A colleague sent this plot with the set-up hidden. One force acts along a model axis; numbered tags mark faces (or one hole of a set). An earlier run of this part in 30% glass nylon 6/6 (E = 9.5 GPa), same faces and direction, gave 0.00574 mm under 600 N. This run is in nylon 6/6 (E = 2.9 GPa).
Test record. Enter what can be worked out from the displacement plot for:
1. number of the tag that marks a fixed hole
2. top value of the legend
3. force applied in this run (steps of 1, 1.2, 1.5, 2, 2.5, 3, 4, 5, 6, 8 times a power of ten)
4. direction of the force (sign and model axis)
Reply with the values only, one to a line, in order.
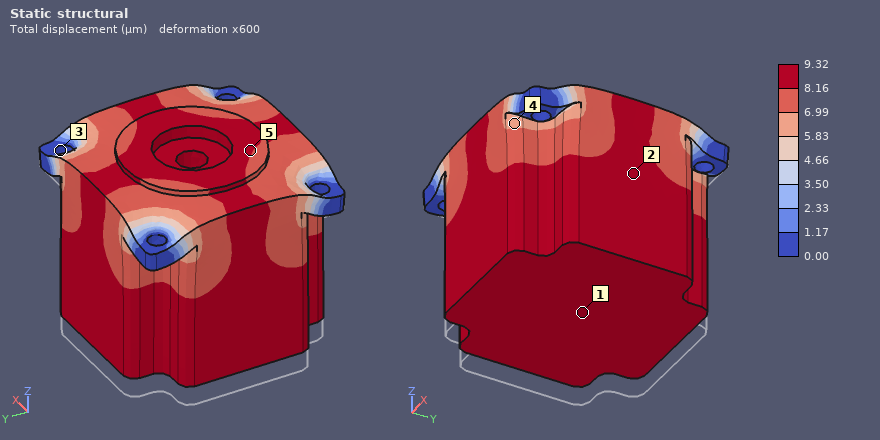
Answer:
3
9.32 µm
300 N
+Z
